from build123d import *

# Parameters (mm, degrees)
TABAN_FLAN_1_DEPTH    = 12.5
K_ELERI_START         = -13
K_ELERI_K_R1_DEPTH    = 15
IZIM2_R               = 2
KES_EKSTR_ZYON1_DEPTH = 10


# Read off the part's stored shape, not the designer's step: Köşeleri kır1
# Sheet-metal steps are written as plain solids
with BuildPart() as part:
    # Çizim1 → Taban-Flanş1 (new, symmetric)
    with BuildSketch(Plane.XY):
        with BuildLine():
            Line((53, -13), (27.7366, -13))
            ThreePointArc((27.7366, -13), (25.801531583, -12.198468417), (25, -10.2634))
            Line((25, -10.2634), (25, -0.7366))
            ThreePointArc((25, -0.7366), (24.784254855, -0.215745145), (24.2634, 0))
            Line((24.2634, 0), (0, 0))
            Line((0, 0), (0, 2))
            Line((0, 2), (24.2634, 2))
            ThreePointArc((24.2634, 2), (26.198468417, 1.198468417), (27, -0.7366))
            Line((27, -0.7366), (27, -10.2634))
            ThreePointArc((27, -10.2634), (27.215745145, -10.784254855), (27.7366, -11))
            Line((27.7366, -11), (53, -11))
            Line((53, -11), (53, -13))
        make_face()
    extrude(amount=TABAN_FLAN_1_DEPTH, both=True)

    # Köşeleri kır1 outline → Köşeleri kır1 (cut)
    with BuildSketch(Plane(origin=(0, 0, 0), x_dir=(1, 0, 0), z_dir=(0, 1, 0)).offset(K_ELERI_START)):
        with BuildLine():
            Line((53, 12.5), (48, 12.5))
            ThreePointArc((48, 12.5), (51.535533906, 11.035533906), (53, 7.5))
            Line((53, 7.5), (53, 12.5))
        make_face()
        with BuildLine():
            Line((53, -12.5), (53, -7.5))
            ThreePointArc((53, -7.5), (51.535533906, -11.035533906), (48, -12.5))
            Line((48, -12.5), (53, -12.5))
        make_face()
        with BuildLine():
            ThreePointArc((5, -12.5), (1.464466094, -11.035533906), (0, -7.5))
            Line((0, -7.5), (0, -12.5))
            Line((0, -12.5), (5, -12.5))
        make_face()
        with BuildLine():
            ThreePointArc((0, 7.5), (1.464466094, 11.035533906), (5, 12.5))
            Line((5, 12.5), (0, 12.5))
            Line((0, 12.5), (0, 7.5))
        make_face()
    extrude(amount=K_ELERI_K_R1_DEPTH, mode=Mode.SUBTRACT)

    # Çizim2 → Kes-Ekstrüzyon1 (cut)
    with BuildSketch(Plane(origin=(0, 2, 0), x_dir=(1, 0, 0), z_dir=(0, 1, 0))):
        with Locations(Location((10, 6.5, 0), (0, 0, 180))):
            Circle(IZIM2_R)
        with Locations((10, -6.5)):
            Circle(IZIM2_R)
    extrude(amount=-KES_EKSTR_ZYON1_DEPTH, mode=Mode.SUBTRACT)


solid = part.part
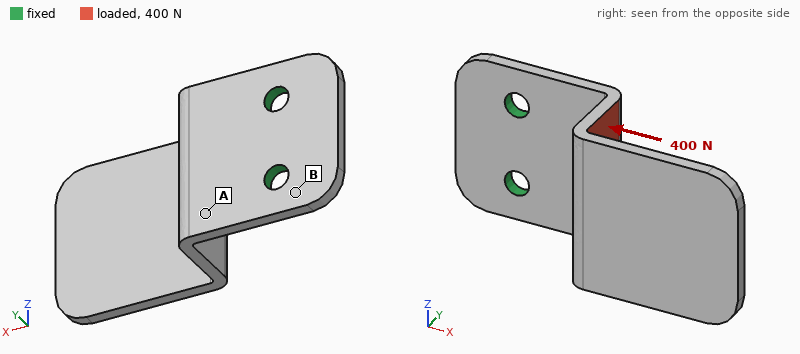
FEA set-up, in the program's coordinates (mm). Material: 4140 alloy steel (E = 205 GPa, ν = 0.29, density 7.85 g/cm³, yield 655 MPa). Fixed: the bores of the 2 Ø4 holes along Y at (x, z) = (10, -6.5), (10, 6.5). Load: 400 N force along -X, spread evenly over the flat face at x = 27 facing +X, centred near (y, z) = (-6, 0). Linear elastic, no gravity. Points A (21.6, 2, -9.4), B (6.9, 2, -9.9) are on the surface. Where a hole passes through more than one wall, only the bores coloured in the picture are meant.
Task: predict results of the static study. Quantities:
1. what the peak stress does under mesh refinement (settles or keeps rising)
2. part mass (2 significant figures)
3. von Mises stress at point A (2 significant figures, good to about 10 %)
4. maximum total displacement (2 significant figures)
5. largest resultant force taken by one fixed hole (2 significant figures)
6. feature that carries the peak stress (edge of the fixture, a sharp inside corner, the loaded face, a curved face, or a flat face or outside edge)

keeps rising
25 g
140 MPa
0.46 mm
200 N
edge of the fixture
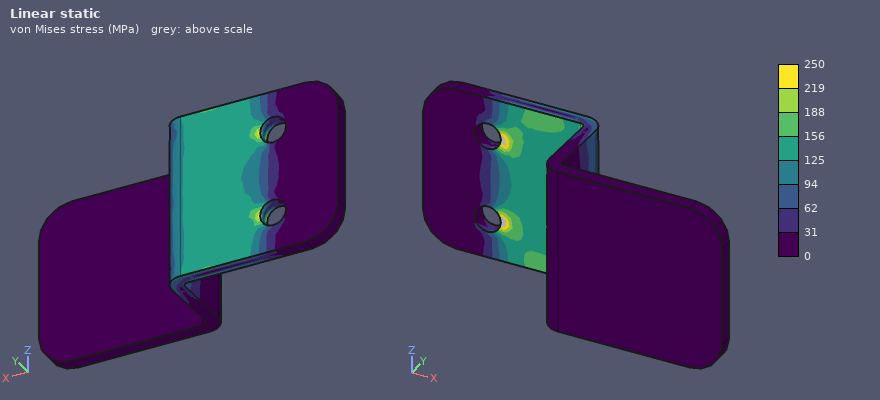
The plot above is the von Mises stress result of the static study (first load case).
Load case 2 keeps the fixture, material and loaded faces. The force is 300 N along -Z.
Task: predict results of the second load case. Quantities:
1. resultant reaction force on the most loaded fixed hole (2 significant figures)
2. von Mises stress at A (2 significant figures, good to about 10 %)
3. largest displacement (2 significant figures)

370 N
47 MPa
52 µm
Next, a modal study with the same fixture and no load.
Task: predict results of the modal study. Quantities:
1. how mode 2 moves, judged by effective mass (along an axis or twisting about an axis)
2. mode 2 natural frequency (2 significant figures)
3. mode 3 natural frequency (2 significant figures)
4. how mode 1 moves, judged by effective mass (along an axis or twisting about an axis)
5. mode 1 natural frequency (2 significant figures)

along Z
2300 Hz
3000 Hz
along Y
760 Hz
